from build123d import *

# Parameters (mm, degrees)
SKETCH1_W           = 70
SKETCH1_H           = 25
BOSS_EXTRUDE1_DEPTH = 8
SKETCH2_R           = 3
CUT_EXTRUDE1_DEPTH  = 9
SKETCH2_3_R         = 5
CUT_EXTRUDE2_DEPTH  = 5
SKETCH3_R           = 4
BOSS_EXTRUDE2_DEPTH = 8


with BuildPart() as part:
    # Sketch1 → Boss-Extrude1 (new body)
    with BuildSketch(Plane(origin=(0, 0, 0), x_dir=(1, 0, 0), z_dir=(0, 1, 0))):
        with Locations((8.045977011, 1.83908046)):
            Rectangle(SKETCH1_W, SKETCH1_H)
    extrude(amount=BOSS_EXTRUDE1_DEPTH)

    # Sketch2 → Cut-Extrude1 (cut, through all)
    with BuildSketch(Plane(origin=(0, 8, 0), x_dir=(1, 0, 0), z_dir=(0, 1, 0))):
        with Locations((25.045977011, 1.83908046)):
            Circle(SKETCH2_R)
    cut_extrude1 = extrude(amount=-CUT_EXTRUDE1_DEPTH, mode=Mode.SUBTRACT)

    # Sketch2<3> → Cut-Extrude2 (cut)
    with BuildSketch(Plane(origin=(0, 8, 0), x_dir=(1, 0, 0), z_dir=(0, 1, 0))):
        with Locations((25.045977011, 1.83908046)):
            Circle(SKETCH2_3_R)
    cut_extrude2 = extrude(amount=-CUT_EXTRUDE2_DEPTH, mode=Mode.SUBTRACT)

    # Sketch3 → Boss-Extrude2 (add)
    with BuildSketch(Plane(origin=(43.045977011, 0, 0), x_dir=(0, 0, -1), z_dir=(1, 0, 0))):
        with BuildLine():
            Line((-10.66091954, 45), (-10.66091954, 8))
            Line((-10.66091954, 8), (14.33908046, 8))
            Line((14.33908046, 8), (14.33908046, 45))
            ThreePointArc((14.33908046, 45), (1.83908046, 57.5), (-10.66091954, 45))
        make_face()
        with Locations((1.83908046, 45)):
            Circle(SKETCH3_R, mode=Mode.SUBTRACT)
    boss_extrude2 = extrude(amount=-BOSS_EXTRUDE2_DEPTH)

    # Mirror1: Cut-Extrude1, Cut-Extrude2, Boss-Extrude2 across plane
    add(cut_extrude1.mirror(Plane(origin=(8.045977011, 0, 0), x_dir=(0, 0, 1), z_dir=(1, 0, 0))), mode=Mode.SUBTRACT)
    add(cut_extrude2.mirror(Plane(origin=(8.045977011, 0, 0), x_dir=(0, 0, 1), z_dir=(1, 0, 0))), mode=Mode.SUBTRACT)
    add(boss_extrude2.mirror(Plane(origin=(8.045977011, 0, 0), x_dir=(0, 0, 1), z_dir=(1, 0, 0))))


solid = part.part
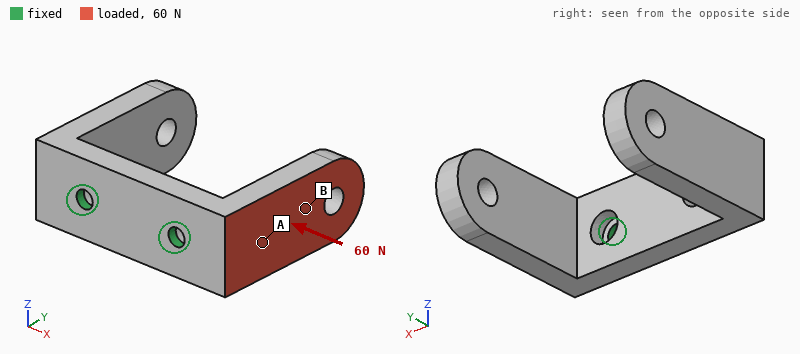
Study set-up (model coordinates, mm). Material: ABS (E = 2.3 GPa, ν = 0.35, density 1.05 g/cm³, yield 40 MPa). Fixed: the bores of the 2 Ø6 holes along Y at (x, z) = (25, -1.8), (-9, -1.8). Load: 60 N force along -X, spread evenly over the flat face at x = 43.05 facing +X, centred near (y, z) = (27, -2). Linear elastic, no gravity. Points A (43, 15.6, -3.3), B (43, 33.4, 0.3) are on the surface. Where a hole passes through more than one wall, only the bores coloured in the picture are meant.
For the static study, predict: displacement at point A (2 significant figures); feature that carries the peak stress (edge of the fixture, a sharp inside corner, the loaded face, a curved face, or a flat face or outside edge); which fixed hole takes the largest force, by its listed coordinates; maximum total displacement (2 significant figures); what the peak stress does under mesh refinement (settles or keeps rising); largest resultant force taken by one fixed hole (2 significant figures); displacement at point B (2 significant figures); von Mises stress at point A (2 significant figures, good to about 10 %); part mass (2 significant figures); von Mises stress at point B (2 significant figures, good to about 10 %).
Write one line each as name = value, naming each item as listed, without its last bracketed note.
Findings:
displacement at point A = 0.25 mm
feature that carries the peak stress = edge of the fixture
which fixed hole takes the largest force, by its listed coordinates = (-9, -1.8)
maximum total displacement = 0.99 mm
what the peak stress does under mesh refinement = keeps rising
largest resultant force taken by one fixed hole = 100 N
displacement at point B = 0.53 mm
von Mises stress at point A = 2.9 MPa
part mass = 33 g
von Mises stress at point B = 0.92 MPa
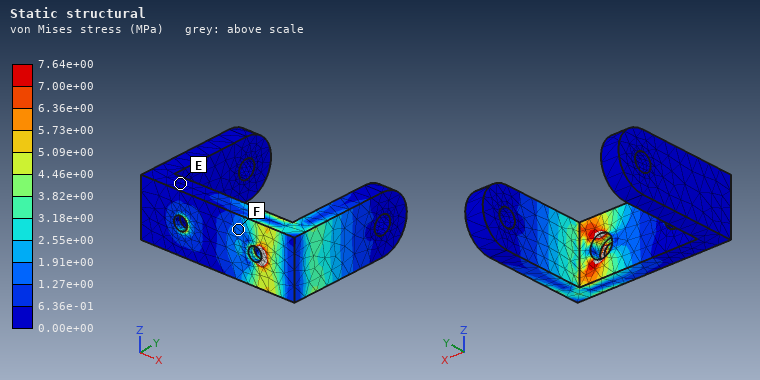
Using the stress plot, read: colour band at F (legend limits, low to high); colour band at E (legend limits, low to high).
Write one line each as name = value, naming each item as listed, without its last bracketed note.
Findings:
colour band at F = 1.27e+00 to 1.91e+00 MPa
colour band at E = 0.00e+00 to 6.36e-01 MPa
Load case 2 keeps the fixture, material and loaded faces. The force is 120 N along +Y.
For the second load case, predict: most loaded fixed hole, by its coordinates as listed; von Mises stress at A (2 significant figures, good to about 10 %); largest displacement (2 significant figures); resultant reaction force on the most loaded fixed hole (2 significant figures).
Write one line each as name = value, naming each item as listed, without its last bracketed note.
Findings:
most loaded fixed hole, by its coordinates as listed = (25, -1.8)
von Mises stress at A = 1.7 MPa
largest displacement = 0.91 mm
resultant reaction force on the most loaded fixed hole = 200 N
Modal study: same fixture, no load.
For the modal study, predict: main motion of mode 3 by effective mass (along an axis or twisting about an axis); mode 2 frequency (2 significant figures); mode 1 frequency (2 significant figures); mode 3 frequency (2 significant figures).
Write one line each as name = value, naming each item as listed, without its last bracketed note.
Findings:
main motion of mode 3 by effective mass = along Z
mode 2 frequency = 470 Hz
mode 1 frequency = 460 Hz
mode 3 frequency = 490 Hz
